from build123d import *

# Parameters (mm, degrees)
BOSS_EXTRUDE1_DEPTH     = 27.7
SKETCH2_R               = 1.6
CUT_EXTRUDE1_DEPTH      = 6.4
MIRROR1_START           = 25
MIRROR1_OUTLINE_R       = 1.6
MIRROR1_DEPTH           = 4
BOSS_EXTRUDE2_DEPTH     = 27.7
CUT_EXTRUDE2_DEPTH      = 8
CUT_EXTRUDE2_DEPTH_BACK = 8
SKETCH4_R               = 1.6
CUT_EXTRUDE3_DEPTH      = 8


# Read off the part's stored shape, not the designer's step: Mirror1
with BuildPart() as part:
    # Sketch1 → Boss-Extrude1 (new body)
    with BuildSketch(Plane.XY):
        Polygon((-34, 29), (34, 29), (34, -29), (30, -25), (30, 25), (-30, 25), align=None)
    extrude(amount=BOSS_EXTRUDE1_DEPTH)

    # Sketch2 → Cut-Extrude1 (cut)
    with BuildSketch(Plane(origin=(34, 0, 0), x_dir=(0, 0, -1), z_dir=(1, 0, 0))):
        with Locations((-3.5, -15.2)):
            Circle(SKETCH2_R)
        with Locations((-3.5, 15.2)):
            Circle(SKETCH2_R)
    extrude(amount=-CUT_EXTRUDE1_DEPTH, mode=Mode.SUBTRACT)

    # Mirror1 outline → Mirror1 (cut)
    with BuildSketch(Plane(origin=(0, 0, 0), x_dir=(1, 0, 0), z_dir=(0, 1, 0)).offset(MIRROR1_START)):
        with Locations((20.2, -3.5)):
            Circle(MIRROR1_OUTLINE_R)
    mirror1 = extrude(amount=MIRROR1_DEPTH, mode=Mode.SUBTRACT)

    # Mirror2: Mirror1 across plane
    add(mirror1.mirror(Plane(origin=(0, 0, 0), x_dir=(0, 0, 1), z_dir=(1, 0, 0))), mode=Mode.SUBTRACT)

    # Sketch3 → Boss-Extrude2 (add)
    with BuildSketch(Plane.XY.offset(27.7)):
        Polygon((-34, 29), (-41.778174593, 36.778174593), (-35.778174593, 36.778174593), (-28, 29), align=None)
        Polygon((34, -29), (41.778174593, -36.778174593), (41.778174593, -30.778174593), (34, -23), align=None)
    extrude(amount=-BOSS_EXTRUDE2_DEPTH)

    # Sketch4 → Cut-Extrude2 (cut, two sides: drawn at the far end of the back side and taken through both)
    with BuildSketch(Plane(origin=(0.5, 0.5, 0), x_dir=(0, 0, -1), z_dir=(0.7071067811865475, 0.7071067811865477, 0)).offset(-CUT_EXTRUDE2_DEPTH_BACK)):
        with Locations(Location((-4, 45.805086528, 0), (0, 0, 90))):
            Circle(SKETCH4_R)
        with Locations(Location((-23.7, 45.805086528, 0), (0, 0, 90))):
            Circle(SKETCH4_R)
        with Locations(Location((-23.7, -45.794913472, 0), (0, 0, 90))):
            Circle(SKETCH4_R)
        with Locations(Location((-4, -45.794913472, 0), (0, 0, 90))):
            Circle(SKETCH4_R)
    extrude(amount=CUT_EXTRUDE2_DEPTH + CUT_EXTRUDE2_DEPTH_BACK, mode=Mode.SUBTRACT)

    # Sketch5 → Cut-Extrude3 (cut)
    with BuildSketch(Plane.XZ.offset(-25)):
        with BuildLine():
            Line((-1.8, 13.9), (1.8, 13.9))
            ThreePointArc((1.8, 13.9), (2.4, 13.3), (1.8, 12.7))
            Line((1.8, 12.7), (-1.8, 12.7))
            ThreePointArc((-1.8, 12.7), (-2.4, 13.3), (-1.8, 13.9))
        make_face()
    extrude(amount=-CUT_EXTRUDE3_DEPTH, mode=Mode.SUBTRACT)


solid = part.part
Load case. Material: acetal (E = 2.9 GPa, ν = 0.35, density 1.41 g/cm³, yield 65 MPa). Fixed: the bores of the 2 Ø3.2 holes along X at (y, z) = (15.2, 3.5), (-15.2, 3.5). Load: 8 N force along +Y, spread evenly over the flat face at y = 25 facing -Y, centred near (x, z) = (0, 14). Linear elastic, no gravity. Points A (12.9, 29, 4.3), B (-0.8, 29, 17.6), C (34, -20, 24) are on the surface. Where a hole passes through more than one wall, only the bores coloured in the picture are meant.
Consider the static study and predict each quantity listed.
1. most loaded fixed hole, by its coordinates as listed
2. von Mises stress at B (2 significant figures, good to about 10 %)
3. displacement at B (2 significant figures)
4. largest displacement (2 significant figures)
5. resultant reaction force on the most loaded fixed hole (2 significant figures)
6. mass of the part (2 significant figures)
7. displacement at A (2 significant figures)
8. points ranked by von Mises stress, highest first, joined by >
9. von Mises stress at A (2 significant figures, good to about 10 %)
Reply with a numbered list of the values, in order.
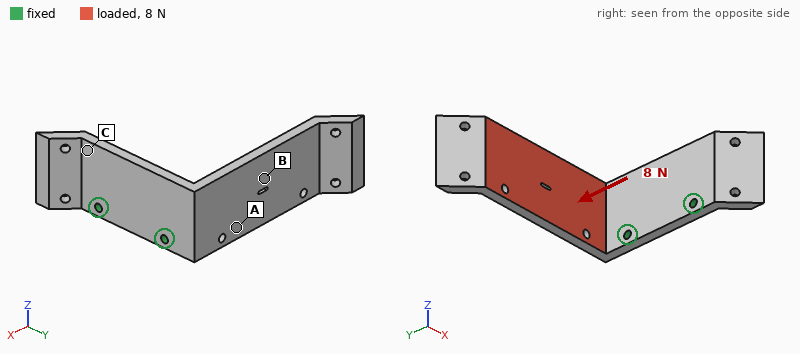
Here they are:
1. (15.2, 3.5)
2. 0.81 MPa
3. 0.49 mm
4. 1.3 mm
5. 7.0 N
6. 22 g
7. 0.25 mm
8. A > B > C
9. 1.6 MPa
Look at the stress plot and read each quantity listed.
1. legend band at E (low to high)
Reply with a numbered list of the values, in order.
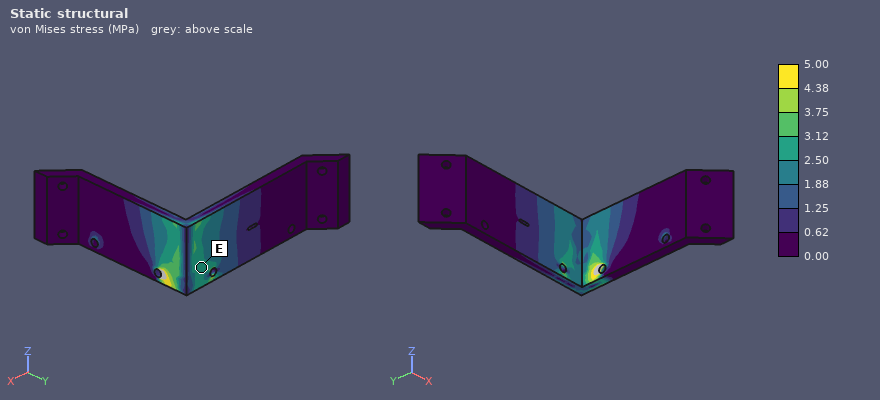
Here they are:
1. 2.50 to 3.12 MPa
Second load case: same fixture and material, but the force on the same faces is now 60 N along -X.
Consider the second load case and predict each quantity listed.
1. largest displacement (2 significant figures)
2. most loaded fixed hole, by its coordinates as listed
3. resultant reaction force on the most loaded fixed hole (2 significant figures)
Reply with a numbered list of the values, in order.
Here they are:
1. 1.1 mm
2. (15.2, 3.5)
3. 68 N
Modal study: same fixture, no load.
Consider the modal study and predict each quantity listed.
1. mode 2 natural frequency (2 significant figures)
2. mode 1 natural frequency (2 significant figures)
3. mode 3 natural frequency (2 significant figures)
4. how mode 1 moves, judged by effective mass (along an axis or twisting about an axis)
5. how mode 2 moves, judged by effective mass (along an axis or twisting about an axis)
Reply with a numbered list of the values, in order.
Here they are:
1. 210 Hz
2. 130 Hz
3. 800 Hz
4. along Y
5. along Z
